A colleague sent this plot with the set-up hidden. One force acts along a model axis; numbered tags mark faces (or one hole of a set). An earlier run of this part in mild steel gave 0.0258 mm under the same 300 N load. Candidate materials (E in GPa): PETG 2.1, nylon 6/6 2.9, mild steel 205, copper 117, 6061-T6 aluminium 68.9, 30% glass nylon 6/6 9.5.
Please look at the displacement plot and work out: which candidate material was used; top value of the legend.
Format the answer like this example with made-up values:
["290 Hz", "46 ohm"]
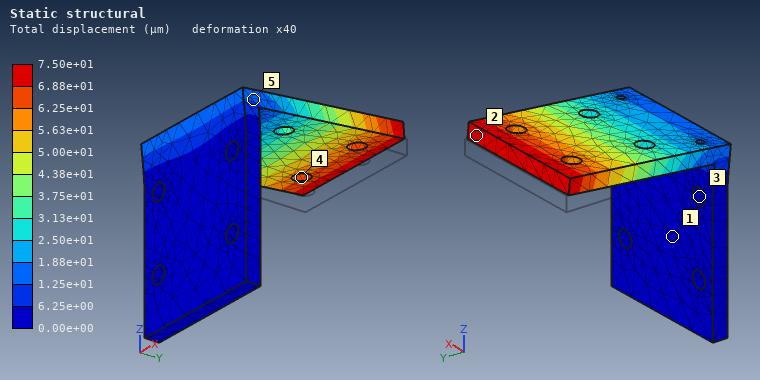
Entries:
["6061-T6 aluminium", "7.50e+01 µm"]
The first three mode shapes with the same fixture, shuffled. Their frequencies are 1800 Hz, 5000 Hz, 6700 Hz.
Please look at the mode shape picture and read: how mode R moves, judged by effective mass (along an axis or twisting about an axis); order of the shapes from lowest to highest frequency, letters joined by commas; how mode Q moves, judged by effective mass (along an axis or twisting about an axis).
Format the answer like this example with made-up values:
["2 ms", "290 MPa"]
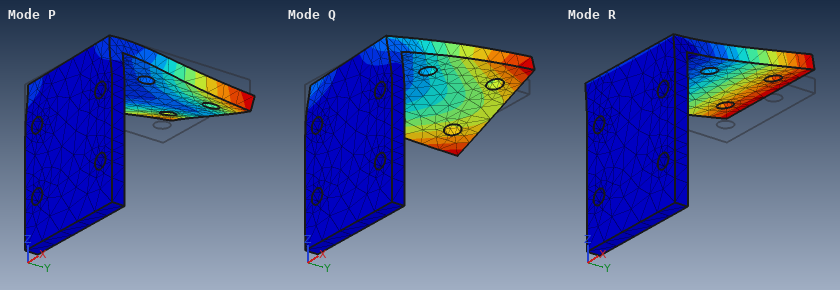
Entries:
["along Z", "R, Q, P", "along X"]
